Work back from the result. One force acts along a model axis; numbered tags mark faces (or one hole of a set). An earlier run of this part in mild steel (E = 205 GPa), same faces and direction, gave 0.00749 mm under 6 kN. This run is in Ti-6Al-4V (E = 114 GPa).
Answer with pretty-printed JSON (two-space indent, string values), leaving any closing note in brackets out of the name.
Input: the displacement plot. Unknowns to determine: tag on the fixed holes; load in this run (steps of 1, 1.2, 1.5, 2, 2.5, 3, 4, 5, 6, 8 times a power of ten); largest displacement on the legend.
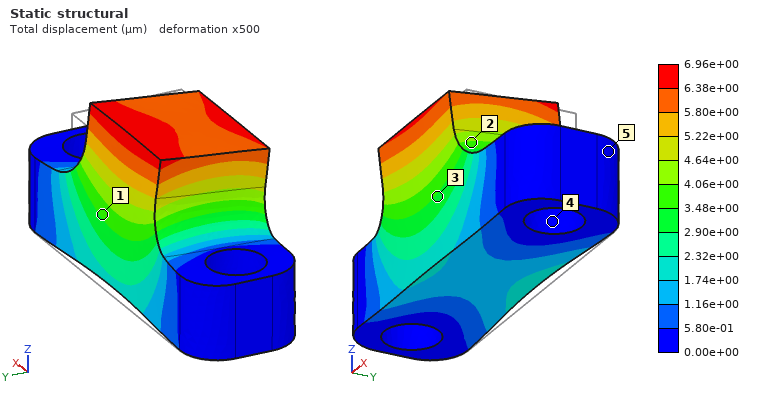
{
  "tag on the fixed holes": "4",
  "load in this run": "3 kN",
  "largest displacement on the legend": "6.96e+00 µm"
}
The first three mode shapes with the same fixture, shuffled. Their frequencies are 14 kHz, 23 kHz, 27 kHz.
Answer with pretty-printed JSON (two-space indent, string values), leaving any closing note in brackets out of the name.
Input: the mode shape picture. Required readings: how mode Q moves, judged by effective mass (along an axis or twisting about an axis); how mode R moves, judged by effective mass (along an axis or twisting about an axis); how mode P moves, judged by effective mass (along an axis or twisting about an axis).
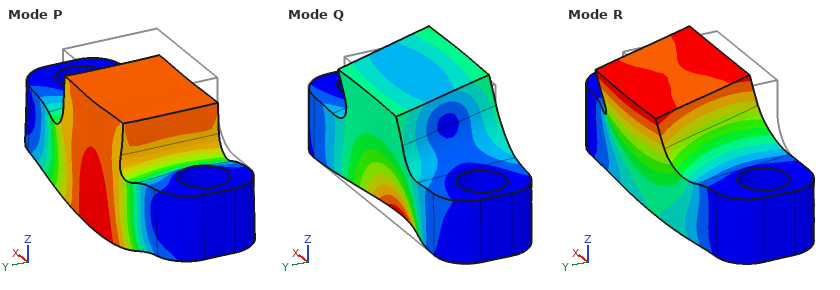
{
  "how mode Q moves, judged by effective mass": "along Y",
  "how mode R moves, judged by effective mass": "along Y",
  "how mode P moves, judged by effective mass": "along Z"
}
